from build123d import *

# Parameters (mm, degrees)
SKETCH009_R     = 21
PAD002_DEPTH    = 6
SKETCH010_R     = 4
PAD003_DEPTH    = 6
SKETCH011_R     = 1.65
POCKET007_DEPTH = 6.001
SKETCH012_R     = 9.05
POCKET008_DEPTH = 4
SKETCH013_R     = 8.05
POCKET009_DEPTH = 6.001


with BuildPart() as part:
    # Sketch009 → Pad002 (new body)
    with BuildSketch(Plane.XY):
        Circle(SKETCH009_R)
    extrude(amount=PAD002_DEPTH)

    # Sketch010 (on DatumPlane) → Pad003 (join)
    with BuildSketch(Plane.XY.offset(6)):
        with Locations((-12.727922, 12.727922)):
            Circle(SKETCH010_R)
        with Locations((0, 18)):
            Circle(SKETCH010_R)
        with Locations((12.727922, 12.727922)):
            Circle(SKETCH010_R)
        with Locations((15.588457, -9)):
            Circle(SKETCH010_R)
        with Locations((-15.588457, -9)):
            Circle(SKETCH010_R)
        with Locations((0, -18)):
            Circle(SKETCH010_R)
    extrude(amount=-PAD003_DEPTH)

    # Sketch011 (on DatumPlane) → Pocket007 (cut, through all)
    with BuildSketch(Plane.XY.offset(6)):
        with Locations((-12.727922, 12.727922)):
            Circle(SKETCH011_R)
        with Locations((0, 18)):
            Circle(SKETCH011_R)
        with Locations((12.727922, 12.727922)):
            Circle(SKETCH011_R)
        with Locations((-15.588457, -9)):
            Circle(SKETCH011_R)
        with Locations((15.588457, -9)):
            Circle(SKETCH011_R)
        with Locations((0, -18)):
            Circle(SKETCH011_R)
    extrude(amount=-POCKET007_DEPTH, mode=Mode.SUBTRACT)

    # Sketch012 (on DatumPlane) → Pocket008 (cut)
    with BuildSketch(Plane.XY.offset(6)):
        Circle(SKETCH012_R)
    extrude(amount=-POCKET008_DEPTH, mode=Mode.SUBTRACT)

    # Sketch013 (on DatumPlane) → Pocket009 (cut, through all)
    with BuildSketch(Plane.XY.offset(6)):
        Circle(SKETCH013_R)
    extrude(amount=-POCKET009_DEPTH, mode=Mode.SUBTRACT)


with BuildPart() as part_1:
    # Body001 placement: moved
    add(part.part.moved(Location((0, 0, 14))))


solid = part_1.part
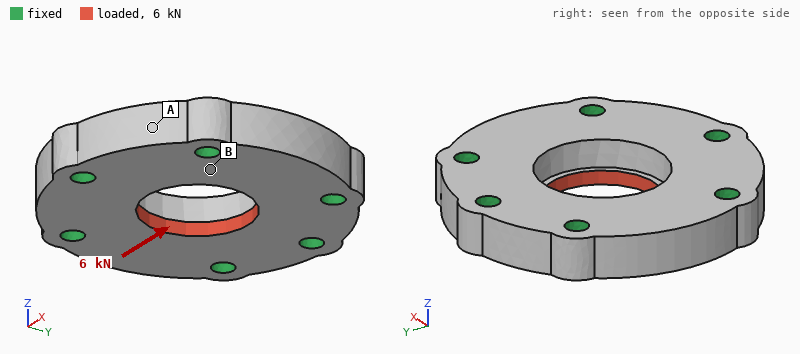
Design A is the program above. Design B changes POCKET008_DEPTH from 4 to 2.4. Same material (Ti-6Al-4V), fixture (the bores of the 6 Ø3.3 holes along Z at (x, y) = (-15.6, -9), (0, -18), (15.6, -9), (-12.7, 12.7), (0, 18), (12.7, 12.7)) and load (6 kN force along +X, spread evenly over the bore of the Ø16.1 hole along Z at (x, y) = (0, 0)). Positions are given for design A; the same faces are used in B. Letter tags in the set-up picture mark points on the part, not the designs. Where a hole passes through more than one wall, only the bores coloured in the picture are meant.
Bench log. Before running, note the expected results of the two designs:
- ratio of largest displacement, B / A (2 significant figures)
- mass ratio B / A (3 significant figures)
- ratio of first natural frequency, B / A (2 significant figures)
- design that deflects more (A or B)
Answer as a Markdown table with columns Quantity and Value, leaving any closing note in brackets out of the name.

| Quantity | Value |
|---|---|
| ratio of largest displacement, B / A | 0.69 |
| mass ratio B / A | 1.01 |
| ratio of first natural frequency, B / A | 0.98 |
| design that deflects more | A |
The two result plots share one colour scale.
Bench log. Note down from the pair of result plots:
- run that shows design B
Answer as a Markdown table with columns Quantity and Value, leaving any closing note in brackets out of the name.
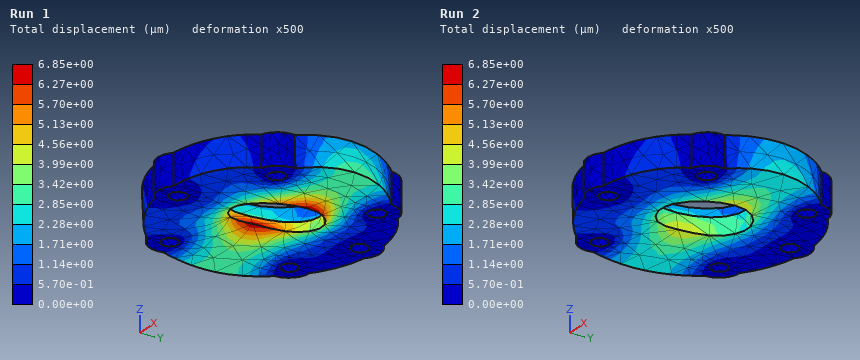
| Quantity | Value |
|---|---|
| run that shows design B | Run 2 |
